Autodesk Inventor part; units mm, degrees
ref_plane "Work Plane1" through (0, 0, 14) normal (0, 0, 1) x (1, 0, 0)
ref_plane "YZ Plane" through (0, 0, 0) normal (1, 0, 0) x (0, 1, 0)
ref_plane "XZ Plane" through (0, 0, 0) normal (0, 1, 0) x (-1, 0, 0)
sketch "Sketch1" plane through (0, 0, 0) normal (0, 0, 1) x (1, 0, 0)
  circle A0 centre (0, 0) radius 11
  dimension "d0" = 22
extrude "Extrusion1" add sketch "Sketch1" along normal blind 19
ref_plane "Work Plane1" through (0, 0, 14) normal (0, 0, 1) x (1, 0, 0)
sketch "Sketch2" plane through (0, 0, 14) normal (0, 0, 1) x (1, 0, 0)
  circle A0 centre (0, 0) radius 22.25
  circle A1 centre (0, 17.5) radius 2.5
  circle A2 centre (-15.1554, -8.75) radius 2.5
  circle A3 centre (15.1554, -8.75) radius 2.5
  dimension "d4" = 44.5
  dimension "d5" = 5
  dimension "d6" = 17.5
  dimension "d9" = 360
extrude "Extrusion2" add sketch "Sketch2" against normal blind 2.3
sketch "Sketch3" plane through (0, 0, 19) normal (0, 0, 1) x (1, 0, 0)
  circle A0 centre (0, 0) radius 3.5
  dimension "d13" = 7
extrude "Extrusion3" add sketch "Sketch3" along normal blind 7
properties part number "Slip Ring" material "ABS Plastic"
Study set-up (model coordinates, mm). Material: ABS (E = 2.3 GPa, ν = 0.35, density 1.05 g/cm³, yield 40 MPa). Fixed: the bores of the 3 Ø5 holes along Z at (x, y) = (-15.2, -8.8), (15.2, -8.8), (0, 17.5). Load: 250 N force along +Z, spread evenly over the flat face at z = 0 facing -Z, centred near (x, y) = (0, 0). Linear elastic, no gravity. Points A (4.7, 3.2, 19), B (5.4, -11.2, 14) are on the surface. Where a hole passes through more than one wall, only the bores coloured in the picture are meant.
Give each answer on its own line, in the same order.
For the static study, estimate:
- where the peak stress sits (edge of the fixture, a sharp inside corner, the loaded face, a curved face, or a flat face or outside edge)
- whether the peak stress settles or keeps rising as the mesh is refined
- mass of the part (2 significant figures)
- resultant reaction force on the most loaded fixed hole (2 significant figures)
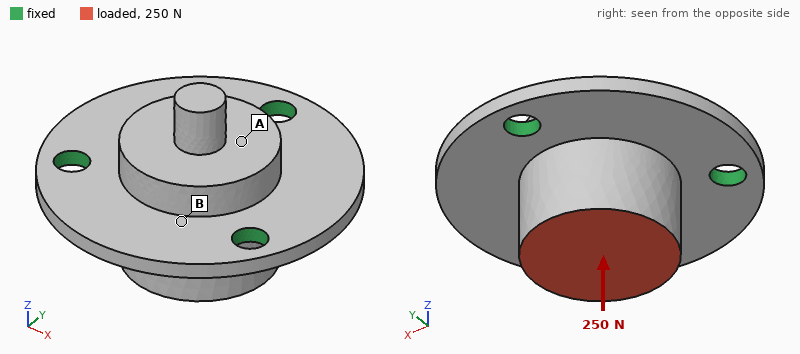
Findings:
edge of the fixture
keeps rising
11 g
83 N
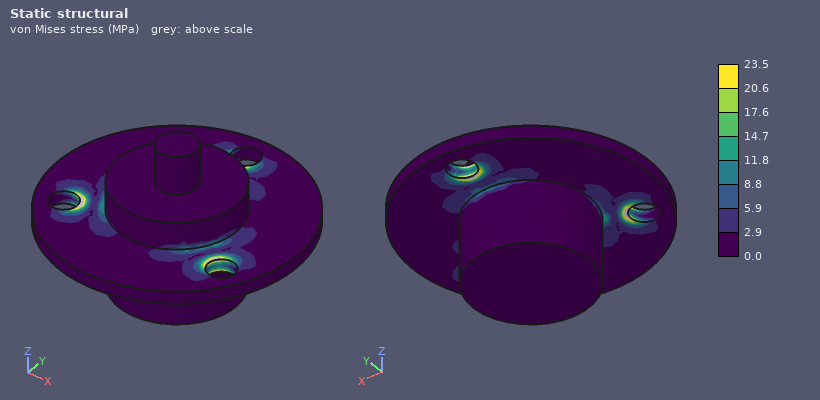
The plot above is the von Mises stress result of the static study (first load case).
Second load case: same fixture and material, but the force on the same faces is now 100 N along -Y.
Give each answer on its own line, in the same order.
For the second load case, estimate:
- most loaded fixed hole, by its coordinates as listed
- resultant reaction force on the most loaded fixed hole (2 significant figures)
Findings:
(0, 17.5)
71 N
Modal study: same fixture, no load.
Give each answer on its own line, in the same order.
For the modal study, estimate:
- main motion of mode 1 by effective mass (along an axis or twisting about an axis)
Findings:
along Z
